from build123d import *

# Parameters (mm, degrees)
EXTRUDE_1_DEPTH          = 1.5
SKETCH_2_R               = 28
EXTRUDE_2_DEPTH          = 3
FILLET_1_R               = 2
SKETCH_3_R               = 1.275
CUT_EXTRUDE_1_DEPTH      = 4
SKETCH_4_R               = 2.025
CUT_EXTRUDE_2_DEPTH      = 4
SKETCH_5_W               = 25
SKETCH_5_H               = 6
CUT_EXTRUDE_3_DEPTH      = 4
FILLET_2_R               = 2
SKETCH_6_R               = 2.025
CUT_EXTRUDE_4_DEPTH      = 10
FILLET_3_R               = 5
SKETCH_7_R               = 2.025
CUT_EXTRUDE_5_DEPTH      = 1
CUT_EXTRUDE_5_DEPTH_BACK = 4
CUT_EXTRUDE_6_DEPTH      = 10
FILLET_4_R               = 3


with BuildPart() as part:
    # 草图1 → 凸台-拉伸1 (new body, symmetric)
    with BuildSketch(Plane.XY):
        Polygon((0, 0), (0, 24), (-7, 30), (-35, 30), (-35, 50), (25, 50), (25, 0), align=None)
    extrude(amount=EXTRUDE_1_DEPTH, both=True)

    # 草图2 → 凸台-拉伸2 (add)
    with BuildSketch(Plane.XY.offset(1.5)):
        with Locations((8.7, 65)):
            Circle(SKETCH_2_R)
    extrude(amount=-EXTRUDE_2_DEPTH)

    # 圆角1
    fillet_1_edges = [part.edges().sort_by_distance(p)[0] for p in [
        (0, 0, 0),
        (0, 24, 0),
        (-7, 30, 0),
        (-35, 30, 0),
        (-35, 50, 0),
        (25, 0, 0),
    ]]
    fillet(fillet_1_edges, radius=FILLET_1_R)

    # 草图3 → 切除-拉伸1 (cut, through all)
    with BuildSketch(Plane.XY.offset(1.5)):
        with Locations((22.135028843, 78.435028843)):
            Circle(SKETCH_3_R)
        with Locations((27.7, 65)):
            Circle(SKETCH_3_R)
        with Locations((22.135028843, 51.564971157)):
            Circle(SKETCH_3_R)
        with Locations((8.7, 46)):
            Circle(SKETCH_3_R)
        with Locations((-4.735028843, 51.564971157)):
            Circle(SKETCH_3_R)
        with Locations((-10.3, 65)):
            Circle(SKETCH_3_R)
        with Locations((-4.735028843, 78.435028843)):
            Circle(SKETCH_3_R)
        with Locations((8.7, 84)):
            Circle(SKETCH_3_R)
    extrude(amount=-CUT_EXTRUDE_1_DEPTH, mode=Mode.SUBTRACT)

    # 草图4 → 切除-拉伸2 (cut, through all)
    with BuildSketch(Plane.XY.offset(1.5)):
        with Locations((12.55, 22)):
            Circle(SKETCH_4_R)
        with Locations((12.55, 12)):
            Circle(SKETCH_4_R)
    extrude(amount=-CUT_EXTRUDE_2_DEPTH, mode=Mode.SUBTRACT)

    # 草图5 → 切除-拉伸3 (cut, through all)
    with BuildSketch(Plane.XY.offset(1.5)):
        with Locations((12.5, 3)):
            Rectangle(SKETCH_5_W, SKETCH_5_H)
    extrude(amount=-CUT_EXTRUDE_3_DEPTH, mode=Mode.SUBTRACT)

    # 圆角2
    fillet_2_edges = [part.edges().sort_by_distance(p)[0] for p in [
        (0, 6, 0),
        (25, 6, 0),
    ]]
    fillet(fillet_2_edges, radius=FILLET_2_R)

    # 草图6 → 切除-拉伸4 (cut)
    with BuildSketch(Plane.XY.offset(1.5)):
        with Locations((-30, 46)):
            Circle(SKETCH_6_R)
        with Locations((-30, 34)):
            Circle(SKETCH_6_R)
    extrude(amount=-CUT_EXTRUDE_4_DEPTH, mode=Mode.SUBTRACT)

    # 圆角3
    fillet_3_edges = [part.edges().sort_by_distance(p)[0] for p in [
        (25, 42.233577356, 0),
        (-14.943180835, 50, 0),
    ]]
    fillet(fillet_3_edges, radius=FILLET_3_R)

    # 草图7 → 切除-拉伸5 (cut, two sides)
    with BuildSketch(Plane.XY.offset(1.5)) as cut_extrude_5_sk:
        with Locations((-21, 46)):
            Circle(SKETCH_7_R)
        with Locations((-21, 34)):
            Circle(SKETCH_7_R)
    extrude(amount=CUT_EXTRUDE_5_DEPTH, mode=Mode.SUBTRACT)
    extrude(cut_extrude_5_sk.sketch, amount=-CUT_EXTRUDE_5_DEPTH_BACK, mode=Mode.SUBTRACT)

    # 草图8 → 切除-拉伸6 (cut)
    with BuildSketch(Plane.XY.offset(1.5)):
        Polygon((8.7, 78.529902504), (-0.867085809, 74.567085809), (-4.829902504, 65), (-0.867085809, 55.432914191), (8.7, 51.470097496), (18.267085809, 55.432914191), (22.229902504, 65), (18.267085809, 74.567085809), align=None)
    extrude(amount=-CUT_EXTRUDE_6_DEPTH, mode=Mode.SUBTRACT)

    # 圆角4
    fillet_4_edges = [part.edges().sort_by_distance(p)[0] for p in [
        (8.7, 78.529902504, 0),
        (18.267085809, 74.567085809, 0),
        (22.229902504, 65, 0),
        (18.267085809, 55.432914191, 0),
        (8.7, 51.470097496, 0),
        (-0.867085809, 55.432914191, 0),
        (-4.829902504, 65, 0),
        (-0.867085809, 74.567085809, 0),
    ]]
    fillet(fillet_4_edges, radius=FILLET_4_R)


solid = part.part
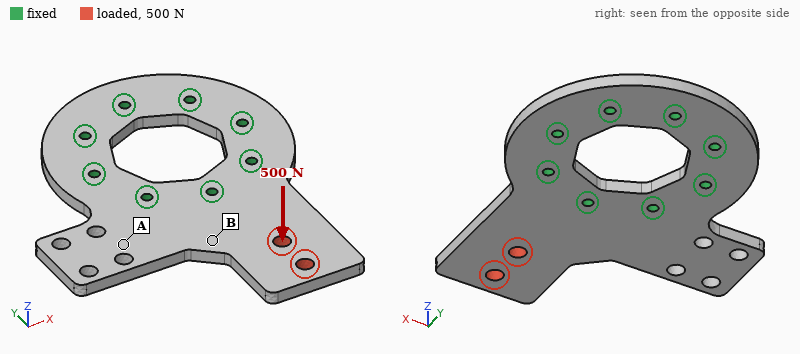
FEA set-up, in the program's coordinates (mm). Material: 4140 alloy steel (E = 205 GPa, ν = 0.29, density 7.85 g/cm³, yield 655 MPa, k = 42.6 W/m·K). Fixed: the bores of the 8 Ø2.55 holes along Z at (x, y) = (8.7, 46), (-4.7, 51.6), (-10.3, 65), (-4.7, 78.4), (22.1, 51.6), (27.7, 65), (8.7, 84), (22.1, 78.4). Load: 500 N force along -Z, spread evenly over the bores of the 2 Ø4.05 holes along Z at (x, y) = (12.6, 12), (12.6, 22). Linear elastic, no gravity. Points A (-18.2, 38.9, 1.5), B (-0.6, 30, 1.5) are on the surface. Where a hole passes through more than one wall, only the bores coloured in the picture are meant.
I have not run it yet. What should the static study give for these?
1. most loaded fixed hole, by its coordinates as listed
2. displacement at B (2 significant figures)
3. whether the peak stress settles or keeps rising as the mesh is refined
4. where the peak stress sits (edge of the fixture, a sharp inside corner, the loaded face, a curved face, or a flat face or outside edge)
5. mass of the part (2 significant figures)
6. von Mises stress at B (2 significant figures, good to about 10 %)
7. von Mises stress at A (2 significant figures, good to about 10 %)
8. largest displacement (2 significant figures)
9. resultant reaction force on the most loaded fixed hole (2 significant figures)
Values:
(8.7, 46)
0.095 mm
keeps rising
edge of the fixture
77 g
180 MPa
47 MPa
0.49 mm
810 N
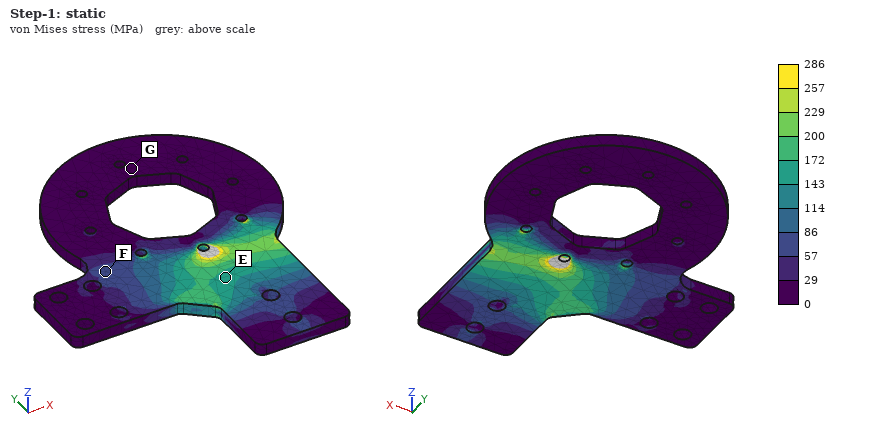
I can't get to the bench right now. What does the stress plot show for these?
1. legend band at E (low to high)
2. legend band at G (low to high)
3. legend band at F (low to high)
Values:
143 to 172 MPa
0 to 29 MPa
57 to 86 MPa
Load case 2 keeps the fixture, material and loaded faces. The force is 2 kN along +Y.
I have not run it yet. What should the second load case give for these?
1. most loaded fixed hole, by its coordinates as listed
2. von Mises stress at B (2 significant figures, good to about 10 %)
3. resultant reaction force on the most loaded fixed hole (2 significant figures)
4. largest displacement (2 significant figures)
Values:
(8.7, 46)
13 MPa
870 N
6.1 µm
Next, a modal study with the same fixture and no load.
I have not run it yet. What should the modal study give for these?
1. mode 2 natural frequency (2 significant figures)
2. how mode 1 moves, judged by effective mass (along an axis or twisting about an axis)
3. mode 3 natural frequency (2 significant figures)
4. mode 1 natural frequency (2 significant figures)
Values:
2600 Hz
along Z
5300 Hz
1700 Hz
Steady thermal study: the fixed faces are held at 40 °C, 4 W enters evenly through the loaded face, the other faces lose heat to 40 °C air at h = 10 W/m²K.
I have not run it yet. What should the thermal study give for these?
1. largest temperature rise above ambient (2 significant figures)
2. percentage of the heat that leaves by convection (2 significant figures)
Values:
34 K
13 %
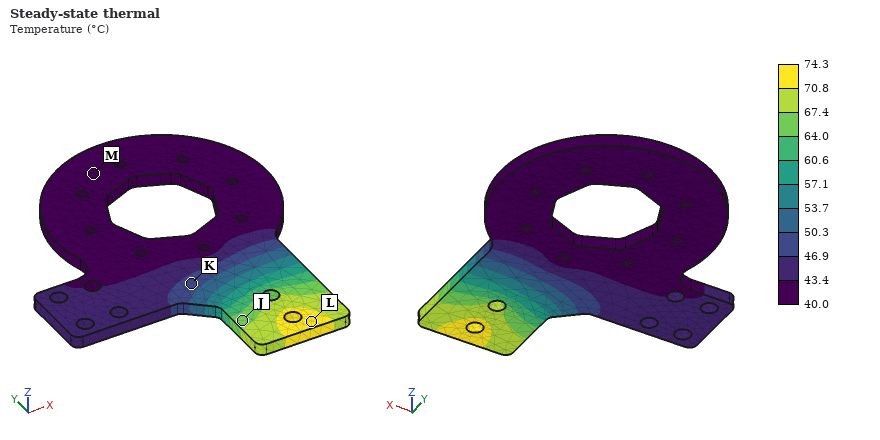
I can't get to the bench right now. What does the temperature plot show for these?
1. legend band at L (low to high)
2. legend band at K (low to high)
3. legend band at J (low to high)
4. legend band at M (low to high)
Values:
70.8 to 74.3 °C
46.9 to 50.3 °C
64.0 to 67.4 °C
40.0 to 43.4 °C
